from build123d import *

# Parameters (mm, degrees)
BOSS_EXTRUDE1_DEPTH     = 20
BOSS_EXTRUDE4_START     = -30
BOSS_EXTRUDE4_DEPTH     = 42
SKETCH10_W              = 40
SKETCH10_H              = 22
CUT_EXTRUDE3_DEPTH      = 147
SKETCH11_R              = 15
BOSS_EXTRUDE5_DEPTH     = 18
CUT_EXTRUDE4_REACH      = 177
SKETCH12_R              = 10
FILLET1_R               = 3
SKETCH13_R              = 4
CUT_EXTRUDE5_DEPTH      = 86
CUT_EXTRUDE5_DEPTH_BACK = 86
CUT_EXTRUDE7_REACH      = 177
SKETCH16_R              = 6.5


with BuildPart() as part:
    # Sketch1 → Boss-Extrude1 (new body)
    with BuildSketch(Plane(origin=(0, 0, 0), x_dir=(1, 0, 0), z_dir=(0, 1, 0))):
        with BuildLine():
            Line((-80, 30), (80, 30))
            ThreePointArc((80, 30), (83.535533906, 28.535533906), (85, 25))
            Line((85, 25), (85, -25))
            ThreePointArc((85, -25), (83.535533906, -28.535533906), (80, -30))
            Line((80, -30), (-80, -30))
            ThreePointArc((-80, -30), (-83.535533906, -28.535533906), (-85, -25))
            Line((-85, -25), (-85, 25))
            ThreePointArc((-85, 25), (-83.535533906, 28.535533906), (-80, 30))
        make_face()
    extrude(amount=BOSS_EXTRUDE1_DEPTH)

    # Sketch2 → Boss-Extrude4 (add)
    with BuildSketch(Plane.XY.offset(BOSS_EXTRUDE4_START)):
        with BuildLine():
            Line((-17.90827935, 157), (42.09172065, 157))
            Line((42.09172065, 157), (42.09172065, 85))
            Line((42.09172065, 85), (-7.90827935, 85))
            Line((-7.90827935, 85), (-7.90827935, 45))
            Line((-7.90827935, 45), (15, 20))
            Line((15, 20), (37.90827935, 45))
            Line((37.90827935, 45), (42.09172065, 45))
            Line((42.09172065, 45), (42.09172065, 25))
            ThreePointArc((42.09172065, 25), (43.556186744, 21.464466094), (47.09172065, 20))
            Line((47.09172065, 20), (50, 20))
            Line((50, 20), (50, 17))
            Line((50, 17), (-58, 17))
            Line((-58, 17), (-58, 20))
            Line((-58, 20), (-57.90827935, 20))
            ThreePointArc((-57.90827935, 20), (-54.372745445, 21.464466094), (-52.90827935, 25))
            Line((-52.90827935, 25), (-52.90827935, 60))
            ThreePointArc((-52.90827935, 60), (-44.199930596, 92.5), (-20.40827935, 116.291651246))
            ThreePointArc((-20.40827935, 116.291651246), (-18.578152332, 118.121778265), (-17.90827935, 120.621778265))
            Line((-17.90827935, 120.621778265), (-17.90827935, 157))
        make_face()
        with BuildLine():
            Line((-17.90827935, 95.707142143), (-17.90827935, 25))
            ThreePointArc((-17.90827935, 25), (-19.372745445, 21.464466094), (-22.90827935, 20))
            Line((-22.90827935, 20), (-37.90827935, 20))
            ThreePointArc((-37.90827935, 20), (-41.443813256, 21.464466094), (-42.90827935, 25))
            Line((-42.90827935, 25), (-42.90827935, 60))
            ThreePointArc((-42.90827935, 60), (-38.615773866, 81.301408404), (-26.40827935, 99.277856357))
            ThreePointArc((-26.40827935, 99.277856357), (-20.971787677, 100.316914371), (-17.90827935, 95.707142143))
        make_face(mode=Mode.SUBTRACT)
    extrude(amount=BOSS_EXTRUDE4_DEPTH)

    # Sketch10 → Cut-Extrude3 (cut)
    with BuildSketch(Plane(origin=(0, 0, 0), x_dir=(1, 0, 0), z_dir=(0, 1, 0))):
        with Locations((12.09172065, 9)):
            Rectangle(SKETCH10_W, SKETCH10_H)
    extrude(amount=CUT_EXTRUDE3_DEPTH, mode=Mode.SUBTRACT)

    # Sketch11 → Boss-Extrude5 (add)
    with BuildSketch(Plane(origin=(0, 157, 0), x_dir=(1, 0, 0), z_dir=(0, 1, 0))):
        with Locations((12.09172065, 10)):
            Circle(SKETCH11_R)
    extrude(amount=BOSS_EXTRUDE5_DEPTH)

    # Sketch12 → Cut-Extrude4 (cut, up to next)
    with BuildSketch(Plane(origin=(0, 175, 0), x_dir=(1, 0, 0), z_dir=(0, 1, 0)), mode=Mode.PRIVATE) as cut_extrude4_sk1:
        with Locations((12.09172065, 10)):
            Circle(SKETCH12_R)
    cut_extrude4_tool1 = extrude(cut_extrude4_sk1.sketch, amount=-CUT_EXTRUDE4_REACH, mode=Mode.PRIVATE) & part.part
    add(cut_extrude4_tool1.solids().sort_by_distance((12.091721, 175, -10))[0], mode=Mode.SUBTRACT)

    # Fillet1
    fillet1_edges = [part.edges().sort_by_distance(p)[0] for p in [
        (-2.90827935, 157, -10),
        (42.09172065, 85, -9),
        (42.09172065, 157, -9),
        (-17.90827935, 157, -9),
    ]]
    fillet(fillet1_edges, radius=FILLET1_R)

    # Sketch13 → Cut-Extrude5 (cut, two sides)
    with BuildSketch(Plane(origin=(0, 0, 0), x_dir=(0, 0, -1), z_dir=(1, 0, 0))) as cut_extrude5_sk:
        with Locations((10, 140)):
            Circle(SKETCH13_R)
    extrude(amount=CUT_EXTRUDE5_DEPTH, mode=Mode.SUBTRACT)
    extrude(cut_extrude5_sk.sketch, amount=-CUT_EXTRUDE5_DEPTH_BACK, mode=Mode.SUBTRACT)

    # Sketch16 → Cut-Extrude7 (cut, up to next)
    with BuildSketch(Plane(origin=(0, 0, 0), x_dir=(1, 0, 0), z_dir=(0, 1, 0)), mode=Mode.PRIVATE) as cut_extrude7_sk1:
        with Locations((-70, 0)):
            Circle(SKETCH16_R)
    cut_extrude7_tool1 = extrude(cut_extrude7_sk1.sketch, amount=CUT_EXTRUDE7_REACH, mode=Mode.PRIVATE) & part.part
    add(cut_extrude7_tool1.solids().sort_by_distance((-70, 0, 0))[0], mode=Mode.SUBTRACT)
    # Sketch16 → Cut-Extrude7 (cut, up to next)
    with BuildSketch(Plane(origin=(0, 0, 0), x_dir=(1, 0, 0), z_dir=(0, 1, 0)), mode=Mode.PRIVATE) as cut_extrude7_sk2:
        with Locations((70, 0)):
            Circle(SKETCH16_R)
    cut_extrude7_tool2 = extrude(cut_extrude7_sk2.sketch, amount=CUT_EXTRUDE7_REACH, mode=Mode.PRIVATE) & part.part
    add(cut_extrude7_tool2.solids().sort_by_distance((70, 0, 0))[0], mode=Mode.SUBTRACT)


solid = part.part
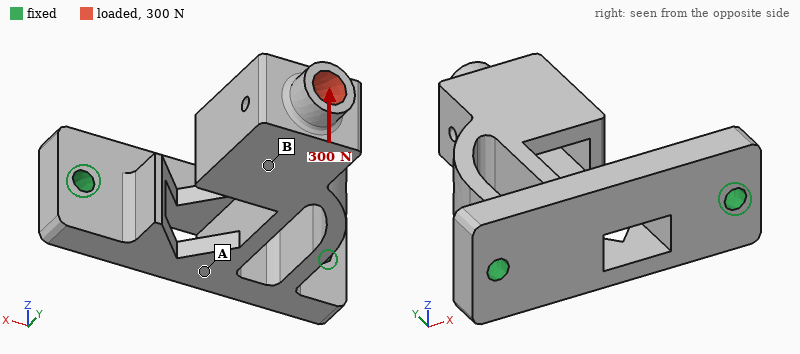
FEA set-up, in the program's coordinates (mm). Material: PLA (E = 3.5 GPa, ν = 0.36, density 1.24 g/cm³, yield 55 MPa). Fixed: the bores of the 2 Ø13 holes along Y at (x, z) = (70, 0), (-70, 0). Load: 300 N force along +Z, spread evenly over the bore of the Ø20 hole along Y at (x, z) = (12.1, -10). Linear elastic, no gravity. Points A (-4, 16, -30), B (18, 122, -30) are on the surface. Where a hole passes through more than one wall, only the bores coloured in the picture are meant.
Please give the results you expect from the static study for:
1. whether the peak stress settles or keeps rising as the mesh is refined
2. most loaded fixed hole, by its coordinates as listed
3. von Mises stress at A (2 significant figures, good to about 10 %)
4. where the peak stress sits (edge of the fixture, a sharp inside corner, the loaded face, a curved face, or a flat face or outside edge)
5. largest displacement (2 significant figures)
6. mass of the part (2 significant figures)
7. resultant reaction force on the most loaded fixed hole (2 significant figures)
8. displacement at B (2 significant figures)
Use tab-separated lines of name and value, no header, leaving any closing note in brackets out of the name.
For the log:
whether the peak stress settles or keeps rising as the mesh is refined	keeps rising
most loaded fixed hole, by its coordinates as listed	(70, 0)
von Mises stress at A	2.7 MPa
where the peak stress sits	edge of the fixture
largest displacement	2.4 mm
mass of the part	500 g
resultant reaction force on the most loaded fixed hole	170 N
displacement at B	1.6 mm
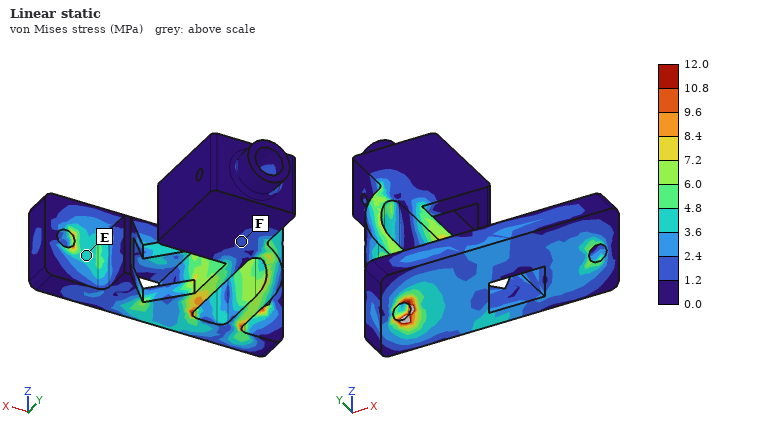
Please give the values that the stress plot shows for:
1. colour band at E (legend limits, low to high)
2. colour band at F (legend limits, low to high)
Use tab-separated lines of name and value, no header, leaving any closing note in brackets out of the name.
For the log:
colour band at E	3.6 to 4.8 MPa
colour band at F	1.2 to 2.4 MPa
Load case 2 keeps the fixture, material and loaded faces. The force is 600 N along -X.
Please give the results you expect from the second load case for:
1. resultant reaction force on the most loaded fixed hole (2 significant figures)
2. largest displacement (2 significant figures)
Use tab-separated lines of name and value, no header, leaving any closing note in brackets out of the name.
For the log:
resultant reaction force on the most loaded fixed hole	780 N
largest displacement	2.7 mm
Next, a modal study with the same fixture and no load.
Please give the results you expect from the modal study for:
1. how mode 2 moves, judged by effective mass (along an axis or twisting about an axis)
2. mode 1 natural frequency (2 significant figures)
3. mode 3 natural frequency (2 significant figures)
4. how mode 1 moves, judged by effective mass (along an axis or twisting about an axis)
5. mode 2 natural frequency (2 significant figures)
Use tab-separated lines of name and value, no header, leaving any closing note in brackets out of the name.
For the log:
how mode 2 moves, judged by effective mass	along X
mode 1 natural frequency	180 Hz
mode 3 natural frequency	550 Hz
how mode 1 moves, judged by effective mass	along Z
mode 2 natural frequency	250 Hz
